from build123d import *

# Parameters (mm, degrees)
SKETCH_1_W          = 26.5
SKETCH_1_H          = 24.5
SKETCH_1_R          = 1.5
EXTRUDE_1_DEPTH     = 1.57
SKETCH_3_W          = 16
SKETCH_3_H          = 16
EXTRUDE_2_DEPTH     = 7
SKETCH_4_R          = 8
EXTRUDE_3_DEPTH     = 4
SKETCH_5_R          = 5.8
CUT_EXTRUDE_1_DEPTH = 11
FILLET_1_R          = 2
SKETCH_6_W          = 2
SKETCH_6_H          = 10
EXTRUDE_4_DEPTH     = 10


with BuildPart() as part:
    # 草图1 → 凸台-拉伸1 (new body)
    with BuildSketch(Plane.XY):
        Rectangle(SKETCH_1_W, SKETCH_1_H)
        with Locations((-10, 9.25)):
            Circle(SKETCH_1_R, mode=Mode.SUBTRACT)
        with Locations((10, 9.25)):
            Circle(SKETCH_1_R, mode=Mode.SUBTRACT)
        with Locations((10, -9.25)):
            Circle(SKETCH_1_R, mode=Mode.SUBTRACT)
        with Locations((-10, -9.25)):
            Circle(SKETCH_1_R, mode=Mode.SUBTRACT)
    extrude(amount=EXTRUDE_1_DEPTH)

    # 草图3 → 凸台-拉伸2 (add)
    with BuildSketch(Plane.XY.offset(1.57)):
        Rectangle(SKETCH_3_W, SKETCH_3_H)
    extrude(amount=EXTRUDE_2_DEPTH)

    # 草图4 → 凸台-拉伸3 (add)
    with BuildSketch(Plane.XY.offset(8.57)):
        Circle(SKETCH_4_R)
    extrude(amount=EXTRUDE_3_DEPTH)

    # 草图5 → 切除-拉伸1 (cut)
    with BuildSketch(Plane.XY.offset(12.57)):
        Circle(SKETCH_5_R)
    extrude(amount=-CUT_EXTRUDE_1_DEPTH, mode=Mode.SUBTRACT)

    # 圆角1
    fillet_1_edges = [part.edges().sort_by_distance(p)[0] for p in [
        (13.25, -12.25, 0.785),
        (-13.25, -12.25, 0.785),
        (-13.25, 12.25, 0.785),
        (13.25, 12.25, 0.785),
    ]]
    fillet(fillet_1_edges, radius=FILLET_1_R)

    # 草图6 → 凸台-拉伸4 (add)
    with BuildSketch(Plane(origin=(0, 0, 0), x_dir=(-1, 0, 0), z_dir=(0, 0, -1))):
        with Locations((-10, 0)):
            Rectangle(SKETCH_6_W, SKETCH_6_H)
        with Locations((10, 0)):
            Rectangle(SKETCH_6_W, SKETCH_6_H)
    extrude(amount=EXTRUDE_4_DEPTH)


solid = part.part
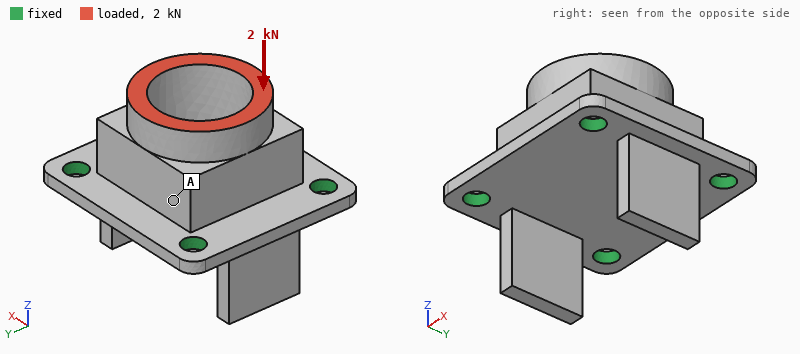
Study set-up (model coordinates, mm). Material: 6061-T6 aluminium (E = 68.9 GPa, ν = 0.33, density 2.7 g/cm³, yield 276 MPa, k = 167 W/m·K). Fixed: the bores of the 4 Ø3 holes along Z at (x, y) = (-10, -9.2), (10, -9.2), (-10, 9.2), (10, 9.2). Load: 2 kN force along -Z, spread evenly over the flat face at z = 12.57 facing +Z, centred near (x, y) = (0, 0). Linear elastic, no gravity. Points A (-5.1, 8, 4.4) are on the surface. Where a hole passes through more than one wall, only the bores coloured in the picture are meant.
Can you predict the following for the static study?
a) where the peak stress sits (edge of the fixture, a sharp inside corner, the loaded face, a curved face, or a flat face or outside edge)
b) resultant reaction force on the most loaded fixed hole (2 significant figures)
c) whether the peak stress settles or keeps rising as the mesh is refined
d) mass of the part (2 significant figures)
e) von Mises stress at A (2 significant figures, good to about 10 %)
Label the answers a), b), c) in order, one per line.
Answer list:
a) edge of the fixture
b) 540 N
c) keeps rising
d) 7.6 g
e) 36 MPa
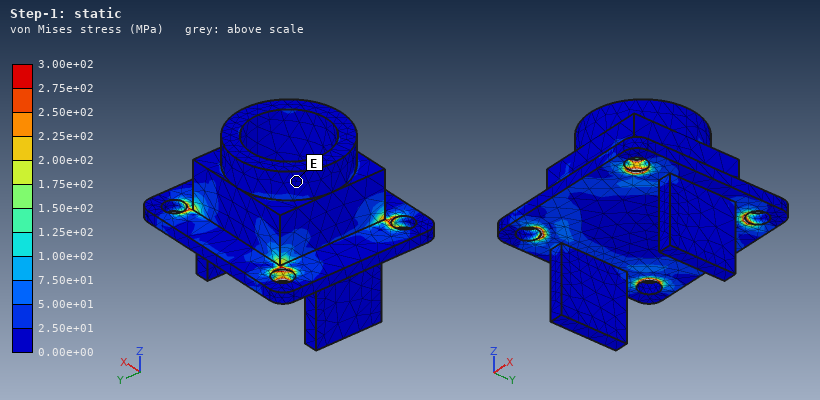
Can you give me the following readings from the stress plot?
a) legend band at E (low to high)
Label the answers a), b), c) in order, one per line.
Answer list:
a) 0.00e+00 to 2.50e+01 MPa
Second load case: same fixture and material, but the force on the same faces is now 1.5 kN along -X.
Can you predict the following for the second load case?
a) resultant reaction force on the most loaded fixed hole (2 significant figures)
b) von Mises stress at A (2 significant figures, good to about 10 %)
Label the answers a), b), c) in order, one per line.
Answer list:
a) 660 N
b) 38 MPa
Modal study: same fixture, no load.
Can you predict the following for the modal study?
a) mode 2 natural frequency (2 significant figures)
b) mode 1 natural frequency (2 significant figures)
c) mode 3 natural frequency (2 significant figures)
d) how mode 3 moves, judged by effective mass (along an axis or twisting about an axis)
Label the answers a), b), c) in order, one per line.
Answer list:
a) 11 kHz
b) 11 kHz
c) 23 kHz
d) along Z
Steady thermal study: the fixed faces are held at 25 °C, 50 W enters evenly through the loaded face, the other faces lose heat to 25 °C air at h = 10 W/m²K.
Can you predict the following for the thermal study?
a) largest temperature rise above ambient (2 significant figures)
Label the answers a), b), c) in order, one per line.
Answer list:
a) 49 K
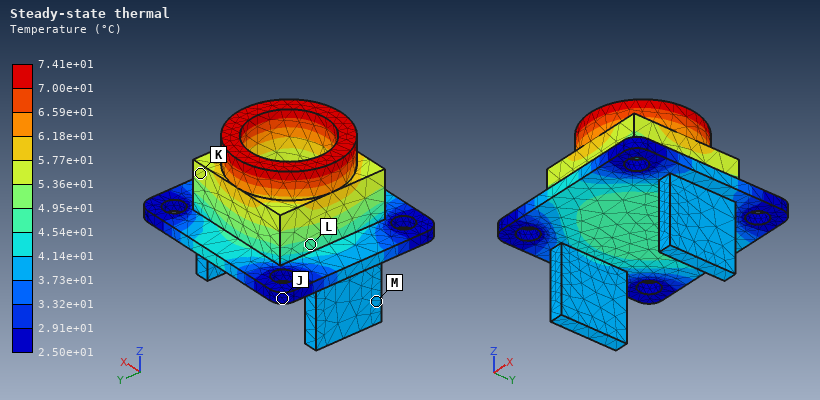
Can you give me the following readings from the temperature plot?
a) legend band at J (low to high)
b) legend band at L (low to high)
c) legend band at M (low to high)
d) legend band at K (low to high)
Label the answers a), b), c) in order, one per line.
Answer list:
a) 2.50e+01 to 2.91e+01 °C
b) 4.54e+01 to 4.95e+01 °C
c) 3.73e+01 to 4.14e+01 °C
d) 5.36e+01 to 5.77e+01 °C
